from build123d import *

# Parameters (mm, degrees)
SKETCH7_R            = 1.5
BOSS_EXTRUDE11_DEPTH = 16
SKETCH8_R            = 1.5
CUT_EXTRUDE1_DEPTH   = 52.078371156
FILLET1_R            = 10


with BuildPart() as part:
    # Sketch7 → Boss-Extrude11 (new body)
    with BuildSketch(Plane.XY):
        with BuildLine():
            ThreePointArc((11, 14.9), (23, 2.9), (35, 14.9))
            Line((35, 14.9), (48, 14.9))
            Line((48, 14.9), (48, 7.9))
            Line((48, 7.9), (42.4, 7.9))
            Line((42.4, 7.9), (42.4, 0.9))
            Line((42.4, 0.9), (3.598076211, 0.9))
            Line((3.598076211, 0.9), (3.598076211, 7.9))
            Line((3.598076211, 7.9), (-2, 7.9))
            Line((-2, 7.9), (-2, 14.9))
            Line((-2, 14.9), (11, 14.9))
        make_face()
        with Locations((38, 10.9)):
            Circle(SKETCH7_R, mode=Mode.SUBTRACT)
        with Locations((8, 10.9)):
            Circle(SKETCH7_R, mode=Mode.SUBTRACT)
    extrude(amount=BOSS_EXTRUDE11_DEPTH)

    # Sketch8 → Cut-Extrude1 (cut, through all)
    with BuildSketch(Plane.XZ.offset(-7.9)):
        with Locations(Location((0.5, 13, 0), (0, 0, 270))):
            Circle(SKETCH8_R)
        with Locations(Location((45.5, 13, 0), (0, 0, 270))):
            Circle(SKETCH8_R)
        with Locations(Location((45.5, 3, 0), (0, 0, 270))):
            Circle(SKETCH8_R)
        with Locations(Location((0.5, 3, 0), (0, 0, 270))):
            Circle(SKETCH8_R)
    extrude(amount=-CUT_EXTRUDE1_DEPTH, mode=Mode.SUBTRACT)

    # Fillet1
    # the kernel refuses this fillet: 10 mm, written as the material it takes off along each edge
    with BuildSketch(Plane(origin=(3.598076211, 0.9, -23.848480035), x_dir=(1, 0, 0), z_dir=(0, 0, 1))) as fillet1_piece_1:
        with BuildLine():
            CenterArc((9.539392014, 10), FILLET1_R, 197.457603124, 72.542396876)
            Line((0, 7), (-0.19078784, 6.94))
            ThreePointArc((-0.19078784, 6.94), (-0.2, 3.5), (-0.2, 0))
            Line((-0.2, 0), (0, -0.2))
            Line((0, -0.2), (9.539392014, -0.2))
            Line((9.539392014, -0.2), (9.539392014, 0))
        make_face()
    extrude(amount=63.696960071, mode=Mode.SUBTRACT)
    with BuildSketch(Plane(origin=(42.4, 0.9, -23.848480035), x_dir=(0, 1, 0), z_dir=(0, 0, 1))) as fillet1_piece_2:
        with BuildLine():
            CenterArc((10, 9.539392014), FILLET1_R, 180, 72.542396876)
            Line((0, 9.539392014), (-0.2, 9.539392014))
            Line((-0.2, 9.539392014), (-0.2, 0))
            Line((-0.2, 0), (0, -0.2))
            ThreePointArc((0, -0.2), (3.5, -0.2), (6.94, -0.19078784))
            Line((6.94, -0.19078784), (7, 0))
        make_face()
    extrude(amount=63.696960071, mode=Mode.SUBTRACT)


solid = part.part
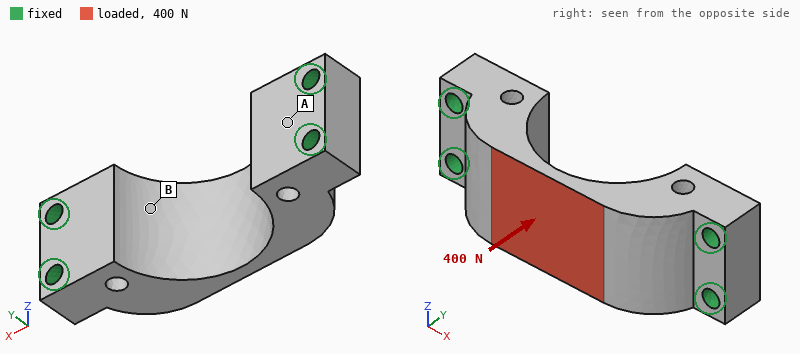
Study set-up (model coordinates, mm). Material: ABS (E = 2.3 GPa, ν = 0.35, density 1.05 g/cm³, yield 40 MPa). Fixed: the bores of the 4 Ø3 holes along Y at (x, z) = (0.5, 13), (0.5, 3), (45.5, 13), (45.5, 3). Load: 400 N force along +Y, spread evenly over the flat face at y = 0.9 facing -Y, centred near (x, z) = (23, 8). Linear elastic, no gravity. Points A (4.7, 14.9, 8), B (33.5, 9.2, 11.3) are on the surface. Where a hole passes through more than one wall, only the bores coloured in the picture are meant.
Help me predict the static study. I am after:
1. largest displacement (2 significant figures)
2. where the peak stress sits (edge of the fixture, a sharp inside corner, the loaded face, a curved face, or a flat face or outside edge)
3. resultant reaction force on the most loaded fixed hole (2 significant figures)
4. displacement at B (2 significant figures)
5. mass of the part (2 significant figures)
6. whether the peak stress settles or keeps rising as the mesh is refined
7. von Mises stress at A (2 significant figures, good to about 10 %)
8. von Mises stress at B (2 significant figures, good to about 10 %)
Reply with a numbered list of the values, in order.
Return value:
1. 0.14 mm
2. edge of the fixture
3. 170 N
4. 0.047 mm
5. 5.6 g
6. keeps rising
7. 2.9 MPa
8. 6.0 MPa
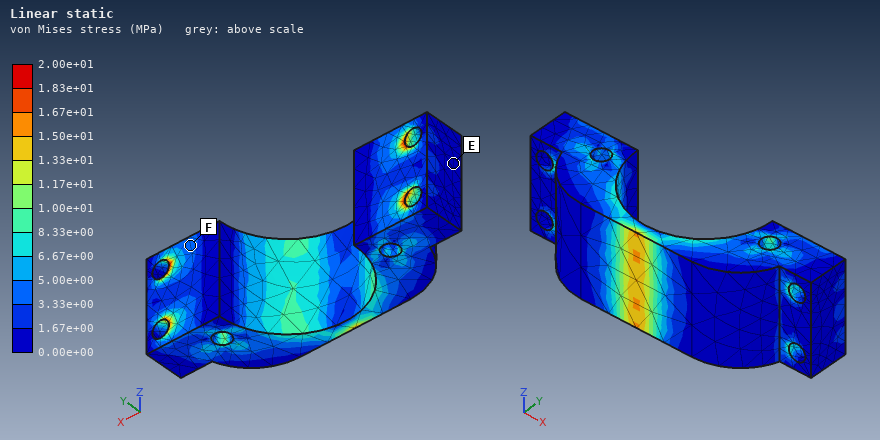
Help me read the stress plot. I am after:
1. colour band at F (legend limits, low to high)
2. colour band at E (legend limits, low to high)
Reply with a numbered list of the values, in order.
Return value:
1. 3.33e+00 to 5.00e+00 MPa
2. 0.00e+00 to 1.67e+00 MPa
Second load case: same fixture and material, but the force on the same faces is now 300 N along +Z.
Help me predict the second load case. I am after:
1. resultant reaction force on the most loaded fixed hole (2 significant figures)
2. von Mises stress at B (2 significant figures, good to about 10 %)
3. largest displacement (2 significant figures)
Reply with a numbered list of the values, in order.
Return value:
1. 220 N
2. 2.1 MPa
3. 0.16 mm
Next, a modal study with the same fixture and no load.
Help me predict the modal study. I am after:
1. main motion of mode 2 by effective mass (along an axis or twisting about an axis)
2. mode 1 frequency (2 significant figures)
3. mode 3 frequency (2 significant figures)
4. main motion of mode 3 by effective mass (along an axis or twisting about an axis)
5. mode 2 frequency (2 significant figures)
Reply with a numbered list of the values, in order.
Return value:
1. along Z
2. 6300 Hz
3. 7800 Hz
4. along Y
5. 6600 Hz
